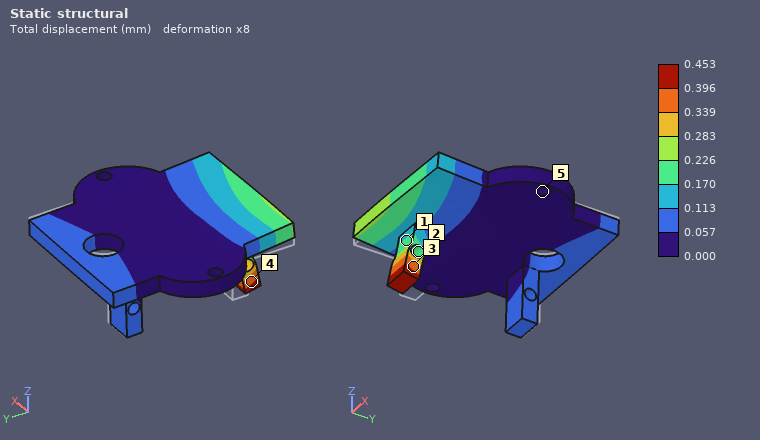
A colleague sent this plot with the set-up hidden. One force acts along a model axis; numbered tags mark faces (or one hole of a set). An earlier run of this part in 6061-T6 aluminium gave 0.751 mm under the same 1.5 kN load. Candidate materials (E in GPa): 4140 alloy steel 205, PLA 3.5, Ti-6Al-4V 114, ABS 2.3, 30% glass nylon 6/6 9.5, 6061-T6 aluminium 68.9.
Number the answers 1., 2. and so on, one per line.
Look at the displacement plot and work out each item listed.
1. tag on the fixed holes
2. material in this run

1. 5
2. Ti-6Al-4V
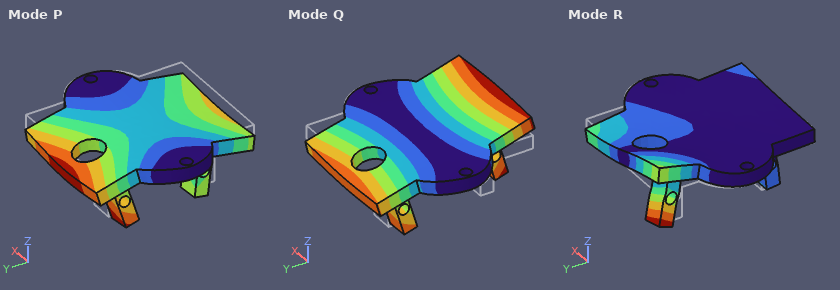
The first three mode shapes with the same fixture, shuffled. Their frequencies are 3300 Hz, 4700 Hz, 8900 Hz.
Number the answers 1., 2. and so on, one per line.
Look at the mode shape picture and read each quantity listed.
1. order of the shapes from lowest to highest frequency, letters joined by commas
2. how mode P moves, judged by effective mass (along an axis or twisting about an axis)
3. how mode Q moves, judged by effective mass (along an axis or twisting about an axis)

1. Q, P, R
2. along Z
3. twisting about X
